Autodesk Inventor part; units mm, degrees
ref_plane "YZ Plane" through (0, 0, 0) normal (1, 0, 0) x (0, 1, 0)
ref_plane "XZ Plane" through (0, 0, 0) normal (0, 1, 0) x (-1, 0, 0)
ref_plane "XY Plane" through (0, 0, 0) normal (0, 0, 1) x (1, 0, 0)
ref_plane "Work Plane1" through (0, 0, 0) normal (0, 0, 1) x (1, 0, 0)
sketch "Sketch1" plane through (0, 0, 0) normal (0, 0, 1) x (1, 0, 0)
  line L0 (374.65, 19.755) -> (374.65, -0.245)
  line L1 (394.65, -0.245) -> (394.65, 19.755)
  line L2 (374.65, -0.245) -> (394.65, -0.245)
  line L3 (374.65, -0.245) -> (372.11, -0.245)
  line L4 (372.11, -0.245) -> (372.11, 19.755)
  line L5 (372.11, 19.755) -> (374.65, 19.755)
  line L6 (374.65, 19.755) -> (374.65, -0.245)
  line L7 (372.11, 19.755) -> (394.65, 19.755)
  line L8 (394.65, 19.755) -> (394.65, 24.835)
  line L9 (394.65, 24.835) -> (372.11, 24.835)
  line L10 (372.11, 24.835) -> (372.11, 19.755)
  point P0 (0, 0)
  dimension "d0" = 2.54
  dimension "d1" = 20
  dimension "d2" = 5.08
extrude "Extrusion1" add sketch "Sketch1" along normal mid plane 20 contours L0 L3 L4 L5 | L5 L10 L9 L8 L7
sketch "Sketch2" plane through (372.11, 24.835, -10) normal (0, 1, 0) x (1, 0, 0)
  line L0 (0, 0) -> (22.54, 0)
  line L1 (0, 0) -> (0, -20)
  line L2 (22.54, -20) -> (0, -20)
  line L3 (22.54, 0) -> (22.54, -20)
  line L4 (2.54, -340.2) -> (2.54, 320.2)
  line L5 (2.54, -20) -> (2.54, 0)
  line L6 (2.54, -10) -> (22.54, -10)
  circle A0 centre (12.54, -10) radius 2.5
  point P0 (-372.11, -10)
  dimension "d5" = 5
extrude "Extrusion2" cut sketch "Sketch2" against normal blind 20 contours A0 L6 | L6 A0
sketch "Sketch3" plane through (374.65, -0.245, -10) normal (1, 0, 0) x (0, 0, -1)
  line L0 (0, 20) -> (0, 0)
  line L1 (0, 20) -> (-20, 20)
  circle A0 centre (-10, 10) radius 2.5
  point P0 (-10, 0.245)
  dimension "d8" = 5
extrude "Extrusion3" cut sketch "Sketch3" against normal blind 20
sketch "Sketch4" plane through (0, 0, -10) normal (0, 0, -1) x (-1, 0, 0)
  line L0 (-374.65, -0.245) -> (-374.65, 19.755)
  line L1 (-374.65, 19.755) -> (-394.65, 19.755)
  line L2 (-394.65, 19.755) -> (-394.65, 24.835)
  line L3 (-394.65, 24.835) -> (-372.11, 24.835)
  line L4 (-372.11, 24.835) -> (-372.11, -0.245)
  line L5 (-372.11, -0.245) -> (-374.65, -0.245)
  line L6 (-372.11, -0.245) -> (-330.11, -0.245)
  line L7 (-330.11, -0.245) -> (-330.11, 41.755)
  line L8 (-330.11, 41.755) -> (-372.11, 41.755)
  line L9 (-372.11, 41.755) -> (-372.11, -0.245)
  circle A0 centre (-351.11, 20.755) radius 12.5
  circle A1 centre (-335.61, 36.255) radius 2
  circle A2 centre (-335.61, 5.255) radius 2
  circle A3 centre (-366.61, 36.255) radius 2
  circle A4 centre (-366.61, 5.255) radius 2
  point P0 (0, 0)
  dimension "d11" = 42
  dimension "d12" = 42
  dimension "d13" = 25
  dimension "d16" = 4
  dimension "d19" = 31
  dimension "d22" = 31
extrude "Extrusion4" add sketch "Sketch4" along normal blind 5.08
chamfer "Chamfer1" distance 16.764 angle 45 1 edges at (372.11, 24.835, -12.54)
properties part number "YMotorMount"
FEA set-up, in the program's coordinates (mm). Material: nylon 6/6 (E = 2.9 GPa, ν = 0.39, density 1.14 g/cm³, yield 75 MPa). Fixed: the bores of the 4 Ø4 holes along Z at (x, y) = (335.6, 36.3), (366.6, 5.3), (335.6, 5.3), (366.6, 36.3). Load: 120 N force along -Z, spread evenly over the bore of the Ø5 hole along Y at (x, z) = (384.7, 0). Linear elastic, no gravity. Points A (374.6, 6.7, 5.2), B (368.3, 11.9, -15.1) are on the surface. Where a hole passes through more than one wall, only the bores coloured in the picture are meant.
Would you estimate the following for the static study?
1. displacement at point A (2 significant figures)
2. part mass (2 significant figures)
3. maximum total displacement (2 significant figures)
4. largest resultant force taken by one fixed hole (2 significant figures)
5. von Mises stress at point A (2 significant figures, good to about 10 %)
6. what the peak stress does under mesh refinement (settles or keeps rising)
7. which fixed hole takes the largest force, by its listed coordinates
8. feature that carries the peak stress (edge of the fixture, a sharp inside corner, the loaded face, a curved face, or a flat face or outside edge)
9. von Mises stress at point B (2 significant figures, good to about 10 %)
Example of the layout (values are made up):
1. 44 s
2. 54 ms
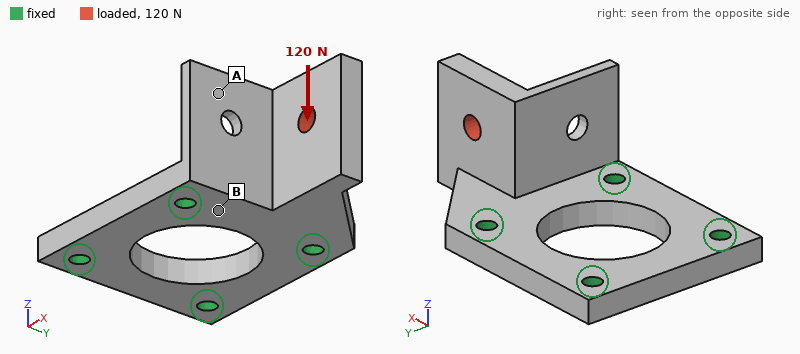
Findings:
1. 0.31 mm
2. 12 g
3. 0.93 mm
4. 80 N
5. 2.5 MPa
6. keeps rising
7. (366.6, 36.3)
8. edge of the fixture
9. 8.0 MPa
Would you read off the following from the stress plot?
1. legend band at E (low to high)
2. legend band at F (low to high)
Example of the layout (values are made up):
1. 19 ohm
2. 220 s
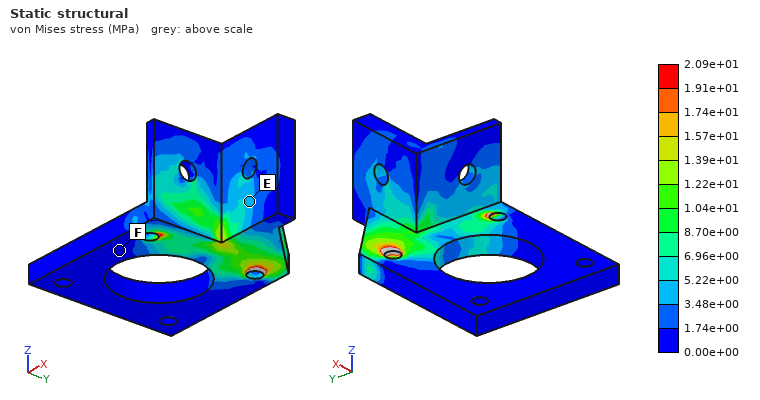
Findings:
1. 3.48e+00 to 5.22e+00 MPa
2. 0.00e+00 to 1.74e+00 MPa
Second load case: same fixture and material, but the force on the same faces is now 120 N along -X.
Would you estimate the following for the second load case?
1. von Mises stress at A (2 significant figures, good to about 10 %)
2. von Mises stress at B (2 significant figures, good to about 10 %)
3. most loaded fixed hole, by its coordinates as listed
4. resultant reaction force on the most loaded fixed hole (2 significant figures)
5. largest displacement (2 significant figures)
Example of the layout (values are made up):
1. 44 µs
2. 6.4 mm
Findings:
1. 2.2 MPa
2. 5.0 MPa
3. (366.6, 36.3)
4. 71 N
5. 0.82 mm
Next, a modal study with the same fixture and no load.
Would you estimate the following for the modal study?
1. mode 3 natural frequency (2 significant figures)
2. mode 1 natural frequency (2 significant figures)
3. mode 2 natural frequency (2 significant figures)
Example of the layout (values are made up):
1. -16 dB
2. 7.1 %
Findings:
1. 2700 Hz
2. 1100 Hz
3. 2300 Hz
